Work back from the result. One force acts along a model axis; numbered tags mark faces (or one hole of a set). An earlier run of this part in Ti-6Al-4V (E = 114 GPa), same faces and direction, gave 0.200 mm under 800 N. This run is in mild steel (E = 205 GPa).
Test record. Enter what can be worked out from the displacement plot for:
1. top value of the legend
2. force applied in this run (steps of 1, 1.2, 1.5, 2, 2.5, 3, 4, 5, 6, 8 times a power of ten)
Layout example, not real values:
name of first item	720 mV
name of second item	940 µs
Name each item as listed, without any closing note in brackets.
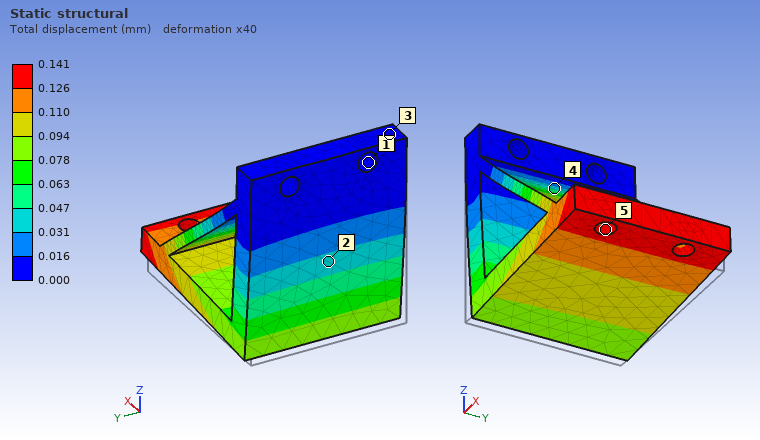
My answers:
top value of the legend	0.141 mm
force applied in this run	1 kN
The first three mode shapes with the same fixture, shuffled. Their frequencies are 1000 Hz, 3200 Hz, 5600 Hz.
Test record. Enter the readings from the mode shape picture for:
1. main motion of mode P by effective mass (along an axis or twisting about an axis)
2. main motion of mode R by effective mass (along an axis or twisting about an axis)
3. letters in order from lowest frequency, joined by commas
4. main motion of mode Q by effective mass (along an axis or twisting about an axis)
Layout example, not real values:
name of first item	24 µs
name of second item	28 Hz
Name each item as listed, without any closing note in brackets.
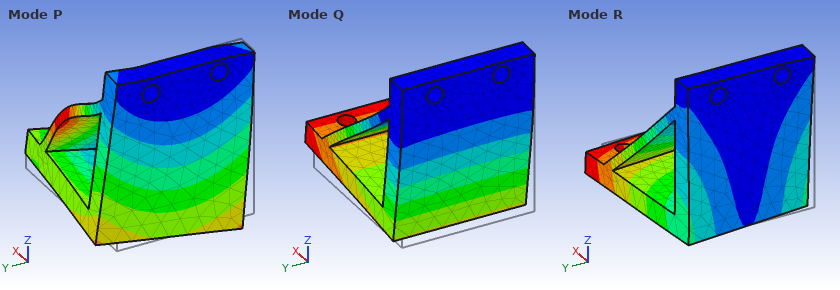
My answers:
main motion of mode P by effective mass	along Y
main motion of mode R by effective mass	along Y
letters in order from lowest frequency, joined by commas	Q, R, P
main motion of mode Q by effective mass	along X
